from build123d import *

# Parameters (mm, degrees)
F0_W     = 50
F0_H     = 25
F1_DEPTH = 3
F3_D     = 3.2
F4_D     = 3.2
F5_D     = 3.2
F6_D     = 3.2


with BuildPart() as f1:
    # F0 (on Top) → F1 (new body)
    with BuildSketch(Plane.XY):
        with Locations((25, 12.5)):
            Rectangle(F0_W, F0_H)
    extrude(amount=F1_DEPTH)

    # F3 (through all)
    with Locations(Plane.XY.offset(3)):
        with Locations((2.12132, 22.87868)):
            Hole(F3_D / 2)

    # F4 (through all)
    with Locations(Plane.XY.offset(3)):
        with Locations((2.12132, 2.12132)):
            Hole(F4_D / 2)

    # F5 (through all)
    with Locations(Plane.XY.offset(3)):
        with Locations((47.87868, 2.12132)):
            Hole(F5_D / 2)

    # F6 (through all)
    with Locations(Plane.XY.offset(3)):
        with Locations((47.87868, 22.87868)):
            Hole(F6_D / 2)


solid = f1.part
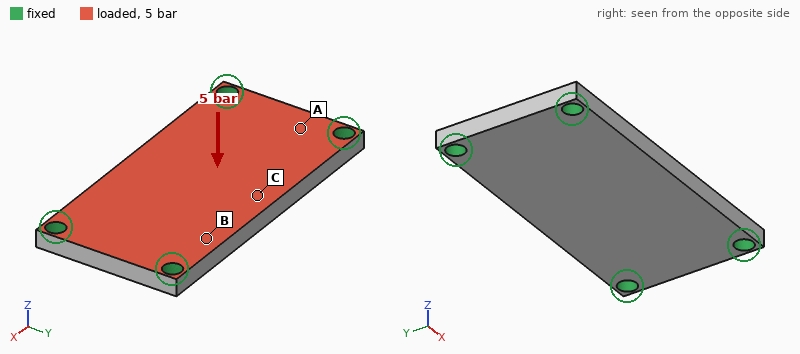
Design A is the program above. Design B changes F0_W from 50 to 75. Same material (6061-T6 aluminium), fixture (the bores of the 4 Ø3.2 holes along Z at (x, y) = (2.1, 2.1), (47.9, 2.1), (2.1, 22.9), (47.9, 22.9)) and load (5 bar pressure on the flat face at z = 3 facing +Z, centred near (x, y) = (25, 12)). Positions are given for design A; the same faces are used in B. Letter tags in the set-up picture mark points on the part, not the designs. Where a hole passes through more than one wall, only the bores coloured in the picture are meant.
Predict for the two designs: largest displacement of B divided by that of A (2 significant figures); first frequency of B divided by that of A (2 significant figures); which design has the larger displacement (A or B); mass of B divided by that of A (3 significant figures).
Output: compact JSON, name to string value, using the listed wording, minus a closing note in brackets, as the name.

{"largest displacement of B divided by that of A": "0.87", "first frequency of B divided by that of A": "1.0", "which design has the larger displacement": "A", "mass of B divided by that of A": "1.51"}
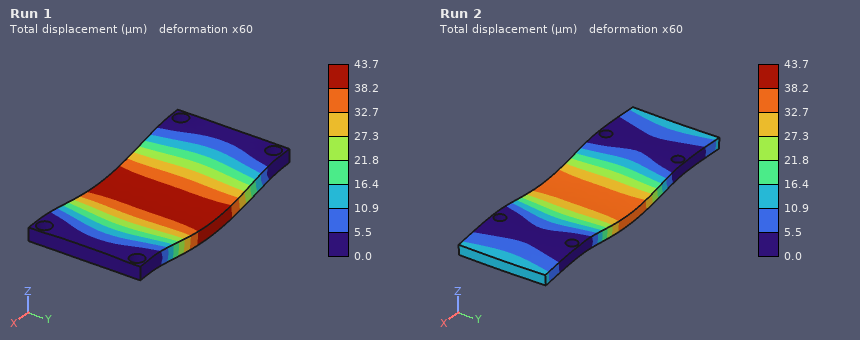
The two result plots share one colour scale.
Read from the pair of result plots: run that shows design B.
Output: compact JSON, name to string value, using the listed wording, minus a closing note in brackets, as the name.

{"run that shows design B": "Run 2"}
